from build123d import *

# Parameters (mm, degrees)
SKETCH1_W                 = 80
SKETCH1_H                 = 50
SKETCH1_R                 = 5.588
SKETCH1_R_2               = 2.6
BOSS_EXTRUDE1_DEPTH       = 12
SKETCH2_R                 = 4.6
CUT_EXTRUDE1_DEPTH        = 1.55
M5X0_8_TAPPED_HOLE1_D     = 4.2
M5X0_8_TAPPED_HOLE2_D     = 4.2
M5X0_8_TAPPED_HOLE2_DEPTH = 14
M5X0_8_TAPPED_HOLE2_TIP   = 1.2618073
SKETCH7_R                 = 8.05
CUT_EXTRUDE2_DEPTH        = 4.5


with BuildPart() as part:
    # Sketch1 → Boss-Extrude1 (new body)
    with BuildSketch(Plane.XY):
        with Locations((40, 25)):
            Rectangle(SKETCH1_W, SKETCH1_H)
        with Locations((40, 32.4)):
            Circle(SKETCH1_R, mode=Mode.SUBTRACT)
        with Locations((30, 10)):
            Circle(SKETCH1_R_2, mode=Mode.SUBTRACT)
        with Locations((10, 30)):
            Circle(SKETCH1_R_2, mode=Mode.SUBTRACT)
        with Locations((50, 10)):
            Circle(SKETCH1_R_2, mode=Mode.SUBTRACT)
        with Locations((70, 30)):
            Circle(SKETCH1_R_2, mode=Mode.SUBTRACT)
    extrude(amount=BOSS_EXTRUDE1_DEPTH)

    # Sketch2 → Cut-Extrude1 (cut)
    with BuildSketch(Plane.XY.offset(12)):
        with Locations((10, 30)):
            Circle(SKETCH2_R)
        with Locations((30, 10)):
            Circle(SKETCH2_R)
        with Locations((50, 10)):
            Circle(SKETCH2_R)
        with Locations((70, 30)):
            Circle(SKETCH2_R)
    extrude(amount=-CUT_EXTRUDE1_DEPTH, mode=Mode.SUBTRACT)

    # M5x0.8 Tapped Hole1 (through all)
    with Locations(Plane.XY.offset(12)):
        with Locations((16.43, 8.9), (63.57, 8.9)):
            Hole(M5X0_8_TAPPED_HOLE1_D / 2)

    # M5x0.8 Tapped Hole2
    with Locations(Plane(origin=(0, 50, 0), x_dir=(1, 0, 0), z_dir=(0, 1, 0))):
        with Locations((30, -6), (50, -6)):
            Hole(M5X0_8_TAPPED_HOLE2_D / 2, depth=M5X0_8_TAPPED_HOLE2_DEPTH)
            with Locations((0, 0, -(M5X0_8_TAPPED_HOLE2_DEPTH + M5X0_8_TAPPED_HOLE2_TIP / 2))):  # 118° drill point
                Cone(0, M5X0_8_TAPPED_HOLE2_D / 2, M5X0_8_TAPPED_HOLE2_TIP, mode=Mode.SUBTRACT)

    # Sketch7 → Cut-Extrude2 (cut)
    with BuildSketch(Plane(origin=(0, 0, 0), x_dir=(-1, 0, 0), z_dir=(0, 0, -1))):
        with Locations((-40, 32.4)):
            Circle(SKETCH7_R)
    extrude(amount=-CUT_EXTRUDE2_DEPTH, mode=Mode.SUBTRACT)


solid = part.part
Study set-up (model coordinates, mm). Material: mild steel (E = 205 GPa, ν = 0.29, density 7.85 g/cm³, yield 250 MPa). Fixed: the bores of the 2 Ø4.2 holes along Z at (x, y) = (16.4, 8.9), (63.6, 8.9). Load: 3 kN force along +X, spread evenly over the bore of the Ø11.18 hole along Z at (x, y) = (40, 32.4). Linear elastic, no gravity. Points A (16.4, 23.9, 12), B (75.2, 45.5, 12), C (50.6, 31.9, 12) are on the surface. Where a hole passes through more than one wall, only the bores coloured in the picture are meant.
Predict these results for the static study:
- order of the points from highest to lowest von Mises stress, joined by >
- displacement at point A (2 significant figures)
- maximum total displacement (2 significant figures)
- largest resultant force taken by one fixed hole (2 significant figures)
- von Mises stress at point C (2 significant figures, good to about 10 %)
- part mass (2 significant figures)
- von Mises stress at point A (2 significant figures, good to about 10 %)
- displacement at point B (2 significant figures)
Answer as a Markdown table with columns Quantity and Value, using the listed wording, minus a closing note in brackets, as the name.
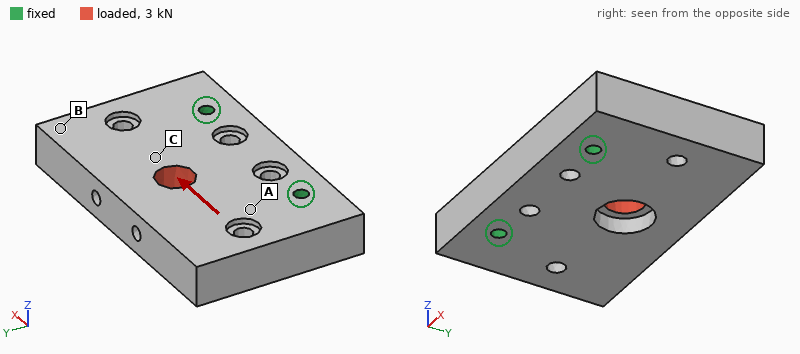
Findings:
| Quantity | Value |
|---|---|
| order of the points from highest to lowest von Mises stress, joined by > | C > A > B |
| displacement at point A | 1.4 µm |
| maximum total displacement | 3.4 µm |
| largest resultant force taken by one fixed hole | 2.0 kN |
| von Mises stress at point C | 14 MPa |
| part mass | 350 g |
| von Mises stress at point A | 5.5 MPa |
| displacement at point B | 3.0 µm |
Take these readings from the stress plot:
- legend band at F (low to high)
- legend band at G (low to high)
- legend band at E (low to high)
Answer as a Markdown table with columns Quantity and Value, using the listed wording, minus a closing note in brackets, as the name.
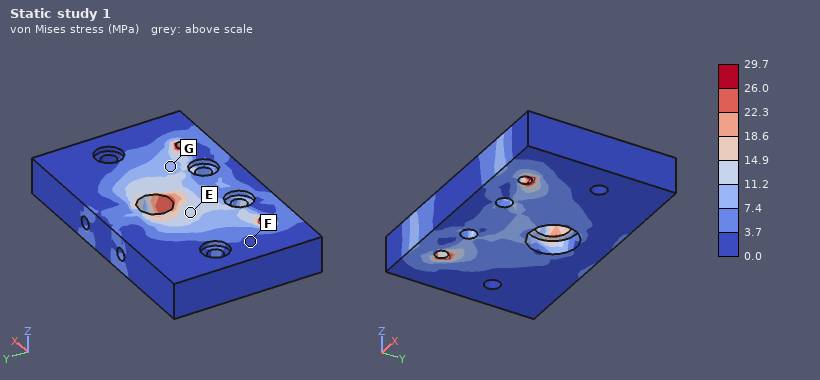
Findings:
| Quantity | Value |
|---|---|
| legend band at F | 0.0 to 3.7 MPa |
| legend band at G | 7.4 to 11.2 MPa |
| legend band at E | 11.2 to 14.9 MPa |
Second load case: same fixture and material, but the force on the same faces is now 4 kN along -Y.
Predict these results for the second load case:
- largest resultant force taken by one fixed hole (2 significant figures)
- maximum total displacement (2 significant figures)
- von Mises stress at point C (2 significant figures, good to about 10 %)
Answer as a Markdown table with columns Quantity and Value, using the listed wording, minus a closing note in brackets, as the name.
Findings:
| Quantity | Value |
|---|---|
| largest resultant force taken by one fixed hole | 2.1 kN |
| maximum total displacement | 5.7 µm |
| von Mises stress at point C | 12 MPa |
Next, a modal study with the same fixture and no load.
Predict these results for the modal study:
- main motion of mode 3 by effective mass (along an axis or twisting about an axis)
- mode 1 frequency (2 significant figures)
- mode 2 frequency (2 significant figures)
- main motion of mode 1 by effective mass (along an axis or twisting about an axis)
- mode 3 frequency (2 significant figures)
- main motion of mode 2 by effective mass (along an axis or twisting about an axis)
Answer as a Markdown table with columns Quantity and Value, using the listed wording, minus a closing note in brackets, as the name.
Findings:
| Quantity | Value |
|---|---|
| main motion of mode 3 by effective mass | along X |
| mode 1 frequency | 4300 Hz |
| mode 2 frequency | 6800 Hz |
| main motion of mode 1 by effective mass | along Z |
| mode 3 frequency | 11 kHz |
| main motion of mode 2 by effective mass | twisting about Y |
